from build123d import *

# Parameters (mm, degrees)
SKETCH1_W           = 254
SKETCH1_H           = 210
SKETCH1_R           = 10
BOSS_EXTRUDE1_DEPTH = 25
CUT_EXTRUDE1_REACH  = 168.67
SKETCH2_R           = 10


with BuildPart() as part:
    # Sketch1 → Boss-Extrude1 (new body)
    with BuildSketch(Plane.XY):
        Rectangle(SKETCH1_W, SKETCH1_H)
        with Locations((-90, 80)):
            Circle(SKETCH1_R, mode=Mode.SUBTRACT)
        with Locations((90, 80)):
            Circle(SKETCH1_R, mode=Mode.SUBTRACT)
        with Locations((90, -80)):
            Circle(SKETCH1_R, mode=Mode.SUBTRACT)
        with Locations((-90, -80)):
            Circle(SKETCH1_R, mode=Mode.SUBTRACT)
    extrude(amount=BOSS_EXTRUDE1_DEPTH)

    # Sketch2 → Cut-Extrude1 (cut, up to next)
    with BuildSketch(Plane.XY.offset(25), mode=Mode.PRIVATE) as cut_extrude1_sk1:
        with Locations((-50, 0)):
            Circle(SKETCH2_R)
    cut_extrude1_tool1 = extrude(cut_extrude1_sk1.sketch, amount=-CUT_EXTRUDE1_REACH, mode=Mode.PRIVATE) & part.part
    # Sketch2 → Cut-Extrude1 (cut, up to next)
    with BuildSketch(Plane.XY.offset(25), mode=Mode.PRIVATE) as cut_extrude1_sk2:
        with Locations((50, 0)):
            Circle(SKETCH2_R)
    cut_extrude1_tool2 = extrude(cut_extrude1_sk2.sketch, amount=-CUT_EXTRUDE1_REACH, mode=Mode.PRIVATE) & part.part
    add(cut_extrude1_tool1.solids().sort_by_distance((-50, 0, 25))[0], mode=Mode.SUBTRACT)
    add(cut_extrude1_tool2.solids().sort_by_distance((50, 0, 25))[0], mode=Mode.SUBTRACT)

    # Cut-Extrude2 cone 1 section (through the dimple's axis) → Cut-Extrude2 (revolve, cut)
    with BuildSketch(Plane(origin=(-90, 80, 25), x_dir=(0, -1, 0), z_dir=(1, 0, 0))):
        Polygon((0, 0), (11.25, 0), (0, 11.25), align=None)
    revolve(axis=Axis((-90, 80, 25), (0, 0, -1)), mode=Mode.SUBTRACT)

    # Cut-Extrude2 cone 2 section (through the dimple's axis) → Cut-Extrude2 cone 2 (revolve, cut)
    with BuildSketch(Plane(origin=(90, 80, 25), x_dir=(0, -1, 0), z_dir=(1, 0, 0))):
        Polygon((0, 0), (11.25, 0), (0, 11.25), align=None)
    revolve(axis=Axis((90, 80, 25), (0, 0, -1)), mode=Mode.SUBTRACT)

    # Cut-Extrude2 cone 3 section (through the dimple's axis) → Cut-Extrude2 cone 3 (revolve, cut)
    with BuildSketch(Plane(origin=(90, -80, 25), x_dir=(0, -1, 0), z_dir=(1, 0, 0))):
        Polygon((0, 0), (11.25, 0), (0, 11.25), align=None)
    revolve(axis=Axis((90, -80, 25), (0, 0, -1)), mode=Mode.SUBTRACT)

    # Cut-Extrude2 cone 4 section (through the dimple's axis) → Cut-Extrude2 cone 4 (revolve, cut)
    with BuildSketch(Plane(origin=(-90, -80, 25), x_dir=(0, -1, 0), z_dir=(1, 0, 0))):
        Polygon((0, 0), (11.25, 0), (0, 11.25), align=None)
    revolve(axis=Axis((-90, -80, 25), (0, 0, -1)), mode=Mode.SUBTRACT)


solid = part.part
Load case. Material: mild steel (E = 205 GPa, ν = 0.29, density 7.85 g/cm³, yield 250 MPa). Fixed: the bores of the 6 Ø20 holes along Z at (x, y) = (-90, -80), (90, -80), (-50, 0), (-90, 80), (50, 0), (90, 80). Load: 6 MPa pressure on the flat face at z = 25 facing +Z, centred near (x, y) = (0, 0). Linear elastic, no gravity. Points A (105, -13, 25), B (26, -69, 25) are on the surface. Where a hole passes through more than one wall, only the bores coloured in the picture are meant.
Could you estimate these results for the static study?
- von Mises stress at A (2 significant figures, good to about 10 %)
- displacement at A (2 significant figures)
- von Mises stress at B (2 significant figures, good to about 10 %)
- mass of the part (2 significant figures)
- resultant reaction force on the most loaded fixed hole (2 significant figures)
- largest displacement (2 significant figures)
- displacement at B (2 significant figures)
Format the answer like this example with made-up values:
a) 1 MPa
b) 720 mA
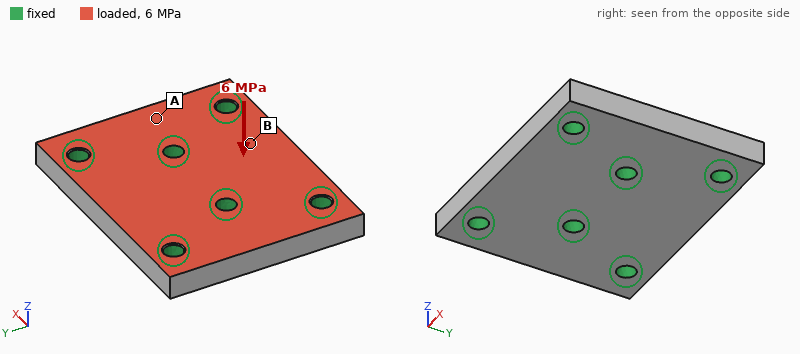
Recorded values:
a) 19 MPa
b) 20 µm
c) 30 MPa
d) 10 kg
e) 62 kN
f) 57 µm
g) 34 µm
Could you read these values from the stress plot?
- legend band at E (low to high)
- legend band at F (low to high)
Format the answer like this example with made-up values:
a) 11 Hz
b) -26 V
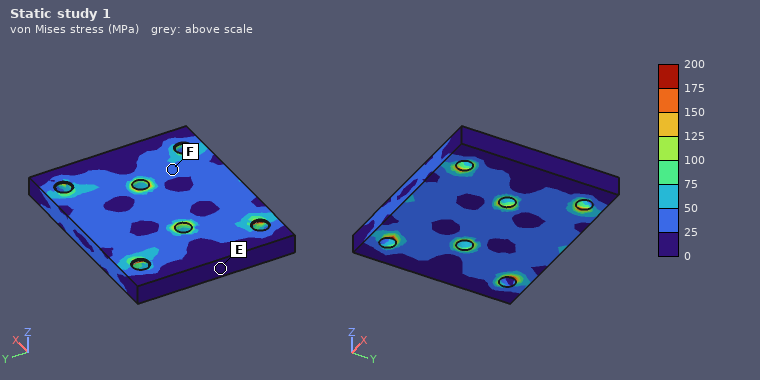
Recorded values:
a) 0 to 25 MPa
b) 25 to 50 MPa
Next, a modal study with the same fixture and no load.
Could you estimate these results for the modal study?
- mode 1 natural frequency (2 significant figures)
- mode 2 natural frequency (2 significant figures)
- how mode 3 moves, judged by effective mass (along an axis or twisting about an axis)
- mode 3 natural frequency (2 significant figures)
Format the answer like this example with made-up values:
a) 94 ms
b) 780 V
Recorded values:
a) 4600 Hz
b) 4700 Hz
c) twisting about Y
d) 6000 Hz
